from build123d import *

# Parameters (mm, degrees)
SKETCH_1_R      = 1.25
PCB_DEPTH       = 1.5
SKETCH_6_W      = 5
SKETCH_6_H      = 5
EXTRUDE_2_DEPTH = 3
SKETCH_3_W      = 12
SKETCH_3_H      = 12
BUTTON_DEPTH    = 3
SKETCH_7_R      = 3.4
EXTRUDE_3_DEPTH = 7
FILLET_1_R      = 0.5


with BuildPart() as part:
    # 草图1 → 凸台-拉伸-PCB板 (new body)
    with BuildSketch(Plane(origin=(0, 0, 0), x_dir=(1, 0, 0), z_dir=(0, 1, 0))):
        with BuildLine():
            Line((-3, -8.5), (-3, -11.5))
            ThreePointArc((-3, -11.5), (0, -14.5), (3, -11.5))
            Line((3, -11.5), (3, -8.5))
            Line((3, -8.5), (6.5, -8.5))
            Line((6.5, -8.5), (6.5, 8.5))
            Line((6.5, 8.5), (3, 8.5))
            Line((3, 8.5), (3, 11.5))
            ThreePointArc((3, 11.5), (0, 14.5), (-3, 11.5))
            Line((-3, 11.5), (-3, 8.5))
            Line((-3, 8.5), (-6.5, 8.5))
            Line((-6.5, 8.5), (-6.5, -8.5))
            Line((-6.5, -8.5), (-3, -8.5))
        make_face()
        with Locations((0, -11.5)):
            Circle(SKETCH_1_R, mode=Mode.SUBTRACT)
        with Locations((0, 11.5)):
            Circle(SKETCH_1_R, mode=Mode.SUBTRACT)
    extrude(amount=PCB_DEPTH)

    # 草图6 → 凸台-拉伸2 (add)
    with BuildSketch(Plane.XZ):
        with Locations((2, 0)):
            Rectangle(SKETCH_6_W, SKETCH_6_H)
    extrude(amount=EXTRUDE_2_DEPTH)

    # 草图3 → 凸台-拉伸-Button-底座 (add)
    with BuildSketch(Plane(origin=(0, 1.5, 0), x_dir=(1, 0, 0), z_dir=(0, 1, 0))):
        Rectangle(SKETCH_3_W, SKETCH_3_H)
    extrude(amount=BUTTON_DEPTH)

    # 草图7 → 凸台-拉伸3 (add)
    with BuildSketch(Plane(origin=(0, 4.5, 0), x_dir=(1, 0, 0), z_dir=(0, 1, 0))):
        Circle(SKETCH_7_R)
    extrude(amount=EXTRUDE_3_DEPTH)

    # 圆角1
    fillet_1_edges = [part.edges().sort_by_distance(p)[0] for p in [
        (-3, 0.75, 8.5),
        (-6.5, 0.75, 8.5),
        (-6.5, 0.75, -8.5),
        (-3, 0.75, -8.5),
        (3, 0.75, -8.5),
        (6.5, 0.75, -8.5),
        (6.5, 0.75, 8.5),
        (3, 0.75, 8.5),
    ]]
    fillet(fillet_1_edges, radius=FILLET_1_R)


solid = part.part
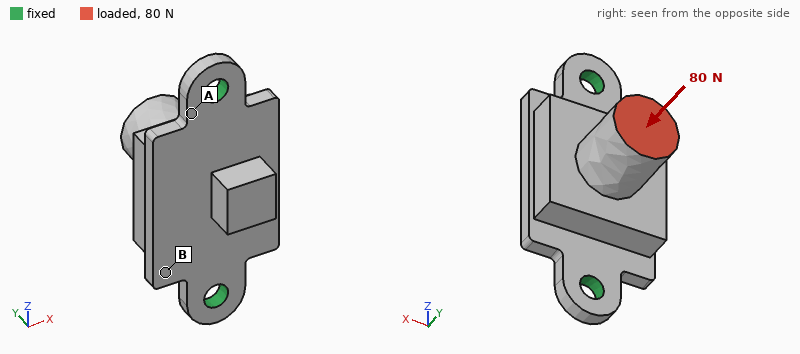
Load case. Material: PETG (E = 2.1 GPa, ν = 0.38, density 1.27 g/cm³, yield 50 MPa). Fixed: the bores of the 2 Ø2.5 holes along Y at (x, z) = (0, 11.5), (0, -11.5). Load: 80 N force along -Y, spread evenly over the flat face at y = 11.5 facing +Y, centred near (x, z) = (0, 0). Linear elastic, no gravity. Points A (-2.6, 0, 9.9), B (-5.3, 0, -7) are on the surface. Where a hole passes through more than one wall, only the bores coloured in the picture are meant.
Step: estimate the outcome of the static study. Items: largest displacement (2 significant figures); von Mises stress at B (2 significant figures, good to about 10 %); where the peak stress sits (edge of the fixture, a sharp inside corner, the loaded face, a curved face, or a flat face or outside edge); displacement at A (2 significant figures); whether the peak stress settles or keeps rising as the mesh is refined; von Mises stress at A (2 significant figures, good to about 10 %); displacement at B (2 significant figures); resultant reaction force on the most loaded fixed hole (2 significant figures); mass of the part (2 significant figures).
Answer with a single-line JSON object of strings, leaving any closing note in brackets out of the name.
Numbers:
{"largest displacement": "0.17 mm", "von Mises stress at B": "7.5 MPa", "where the peak stress sits": "edge of the fixture", "displacement at A": "0.033 mm", "whether the peak stress settles or keeps rising as the mesh is refined": "keeps rising", "von Mises stress at A": "18 MPa", "displacement at B": "0.14 mm", "resultant reaction force on the most loaded fixed hole": "47 N", "mass of the part": "1.5 g"}
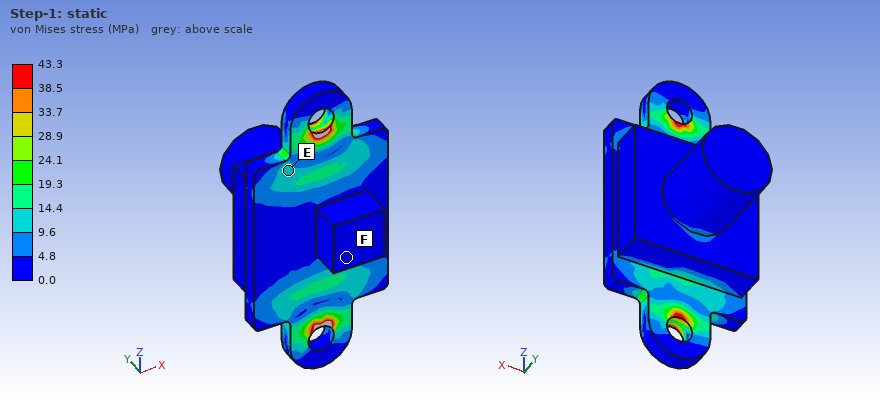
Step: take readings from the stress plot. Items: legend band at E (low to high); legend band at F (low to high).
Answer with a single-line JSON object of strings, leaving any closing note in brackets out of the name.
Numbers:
{"legend band at E": "9.6 to 14.4 MPa", "legend band at F": "0.0 to 4.8 MPa"}
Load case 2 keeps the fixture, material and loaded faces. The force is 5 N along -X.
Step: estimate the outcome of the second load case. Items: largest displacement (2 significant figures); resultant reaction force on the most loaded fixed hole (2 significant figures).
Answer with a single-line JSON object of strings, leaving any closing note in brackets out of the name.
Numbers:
{"largest displacement": "0.20 mm", "resultant reaction force on the most loaded fixed hole": "2.5 N"}
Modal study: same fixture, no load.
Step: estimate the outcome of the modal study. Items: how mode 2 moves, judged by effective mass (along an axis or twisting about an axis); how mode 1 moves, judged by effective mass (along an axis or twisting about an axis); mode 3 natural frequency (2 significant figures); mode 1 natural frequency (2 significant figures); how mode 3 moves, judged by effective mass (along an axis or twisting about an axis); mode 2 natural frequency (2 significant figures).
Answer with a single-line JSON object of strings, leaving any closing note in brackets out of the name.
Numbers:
{"how mode 2 moves, judged by effective mass": "along Y", "how mode 1 moves, judged by effective mass": "along X", "mode 3 natural frequency": "5000 Hz", "mode 1 natural frequency": "1500 Hz", "how mode 3 moves, judged by effective mass": "along Z", "mode 2 natural frequency": "3100 Hz"}
